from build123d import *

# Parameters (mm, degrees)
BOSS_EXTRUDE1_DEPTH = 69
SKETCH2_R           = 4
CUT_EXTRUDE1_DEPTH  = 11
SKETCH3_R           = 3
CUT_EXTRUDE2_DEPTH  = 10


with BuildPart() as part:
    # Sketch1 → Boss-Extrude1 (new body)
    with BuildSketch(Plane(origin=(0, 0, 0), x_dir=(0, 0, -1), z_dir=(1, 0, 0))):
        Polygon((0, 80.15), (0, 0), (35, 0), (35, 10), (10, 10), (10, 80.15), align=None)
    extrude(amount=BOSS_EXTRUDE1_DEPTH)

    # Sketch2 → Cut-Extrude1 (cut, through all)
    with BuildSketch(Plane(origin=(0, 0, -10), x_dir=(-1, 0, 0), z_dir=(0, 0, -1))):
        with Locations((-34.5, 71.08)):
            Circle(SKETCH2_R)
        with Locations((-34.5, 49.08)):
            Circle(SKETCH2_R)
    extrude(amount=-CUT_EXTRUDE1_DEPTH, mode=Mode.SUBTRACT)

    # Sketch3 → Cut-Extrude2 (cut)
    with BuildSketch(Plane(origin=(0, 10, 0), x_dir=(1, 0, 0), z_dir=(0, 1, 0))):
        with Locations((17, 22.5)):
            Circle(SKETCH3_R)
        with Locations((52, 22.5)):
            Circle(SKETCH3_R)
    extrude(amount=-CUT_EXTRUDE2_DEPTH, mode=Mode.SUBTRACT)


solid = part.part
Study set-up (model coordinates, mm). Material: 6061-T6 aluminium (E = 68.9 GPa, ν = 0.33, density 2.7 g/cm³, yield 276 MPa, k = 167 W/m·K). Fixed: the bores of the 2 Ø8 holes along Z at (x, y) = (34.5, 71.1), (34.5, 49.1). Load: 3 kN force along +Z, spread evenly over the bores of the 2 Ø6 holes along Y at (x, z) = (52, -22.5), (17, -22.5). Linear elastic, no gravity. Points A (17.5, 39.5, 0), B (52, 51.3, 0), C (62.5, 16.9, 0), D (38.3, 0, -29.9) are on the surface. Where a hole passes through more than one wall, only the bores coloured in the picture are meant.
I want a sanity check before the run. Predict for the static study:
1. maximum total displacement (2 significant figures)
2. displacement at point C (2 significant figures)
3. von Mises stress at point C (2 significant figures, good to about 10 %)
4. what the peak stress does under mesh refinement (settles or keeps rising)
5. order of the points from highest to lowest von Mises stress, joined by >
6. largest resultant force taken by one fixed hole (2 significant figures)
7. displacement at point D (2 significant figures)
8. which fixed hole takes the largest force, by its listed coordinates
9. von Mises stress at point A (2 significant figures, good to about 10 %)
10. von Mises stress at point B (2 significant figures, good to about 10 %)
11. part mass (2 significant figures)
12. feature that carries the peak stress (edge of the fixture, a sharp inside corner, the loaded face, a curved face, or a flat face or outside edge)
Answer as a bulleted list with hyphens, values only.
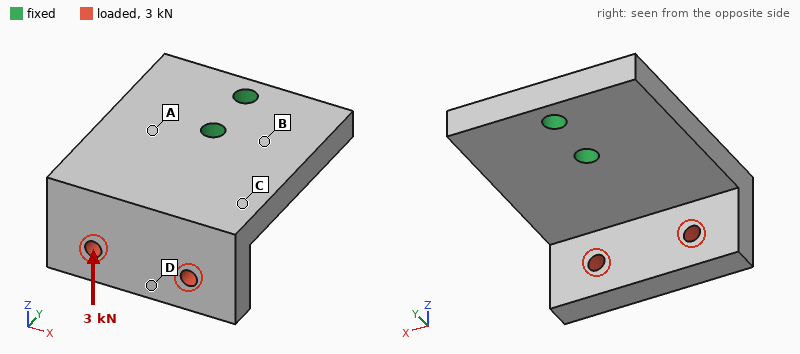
- 0.39 mm
- 0.18 mm
- 30 MPa
- keeps rising
- A > B > C > D
- 5.3 kN
- 0.37 mm
- (34.5, 49.1)
- 73 MPa
- 55 MPa
- 190 g
- edge of the fixture
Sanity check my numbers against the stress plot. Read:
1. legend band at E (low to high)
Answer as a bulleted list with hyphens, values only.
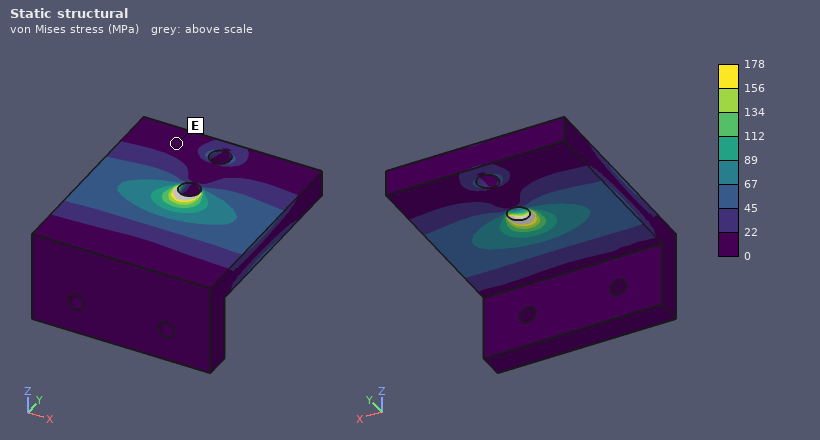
- 0 to 22 MPa
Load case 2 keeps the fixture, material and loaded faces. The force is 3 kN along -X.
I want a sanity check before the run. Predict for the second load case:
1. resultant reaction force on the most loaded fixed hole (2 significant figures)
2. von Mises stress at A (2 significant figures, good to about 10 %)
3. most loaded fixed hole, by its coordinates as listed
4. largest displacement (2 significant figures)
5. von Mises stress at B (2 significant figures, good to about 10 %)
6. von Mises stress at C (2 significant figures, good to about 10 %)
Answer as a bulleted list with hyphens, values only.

- 7.2 kN
- 23 MPa
- (34.5, 49.1)
- 0.20 mm
- 36 MPa
- 19 MPa
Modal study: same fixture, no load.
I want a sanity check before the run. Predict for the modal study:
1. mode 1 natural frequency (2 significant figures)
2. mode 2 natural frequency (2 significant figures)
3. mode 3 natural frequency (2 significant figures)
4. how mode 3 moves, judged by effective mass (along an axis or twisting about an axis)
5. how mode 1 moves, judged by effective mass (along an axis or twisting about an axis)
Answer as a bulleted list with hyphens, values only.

- 1700 Hz
- 2400 Hz
- 4800 Hz
- along X
- along Z
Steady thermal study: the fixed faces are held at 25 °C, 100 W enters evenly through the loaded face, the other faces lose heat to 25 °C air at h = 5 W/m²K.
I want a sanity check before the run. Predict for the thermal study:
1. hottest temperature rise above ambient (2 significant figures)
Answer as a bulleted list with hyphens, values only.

- 62 K
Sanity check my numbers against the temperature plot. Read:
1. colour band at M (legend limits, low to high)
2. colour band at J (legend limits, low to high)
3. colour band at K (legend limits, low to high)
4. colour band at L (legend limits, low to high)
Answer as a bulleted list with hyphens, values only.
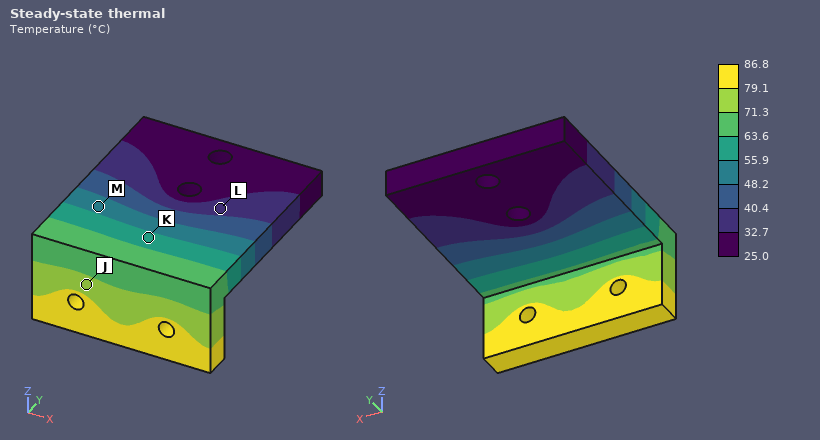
- 48.2 to 55.9 °C
- 71.3 to 79.1 °C
- 55.9 to 63.6 °C
- 32.7 to 40.4 °C
